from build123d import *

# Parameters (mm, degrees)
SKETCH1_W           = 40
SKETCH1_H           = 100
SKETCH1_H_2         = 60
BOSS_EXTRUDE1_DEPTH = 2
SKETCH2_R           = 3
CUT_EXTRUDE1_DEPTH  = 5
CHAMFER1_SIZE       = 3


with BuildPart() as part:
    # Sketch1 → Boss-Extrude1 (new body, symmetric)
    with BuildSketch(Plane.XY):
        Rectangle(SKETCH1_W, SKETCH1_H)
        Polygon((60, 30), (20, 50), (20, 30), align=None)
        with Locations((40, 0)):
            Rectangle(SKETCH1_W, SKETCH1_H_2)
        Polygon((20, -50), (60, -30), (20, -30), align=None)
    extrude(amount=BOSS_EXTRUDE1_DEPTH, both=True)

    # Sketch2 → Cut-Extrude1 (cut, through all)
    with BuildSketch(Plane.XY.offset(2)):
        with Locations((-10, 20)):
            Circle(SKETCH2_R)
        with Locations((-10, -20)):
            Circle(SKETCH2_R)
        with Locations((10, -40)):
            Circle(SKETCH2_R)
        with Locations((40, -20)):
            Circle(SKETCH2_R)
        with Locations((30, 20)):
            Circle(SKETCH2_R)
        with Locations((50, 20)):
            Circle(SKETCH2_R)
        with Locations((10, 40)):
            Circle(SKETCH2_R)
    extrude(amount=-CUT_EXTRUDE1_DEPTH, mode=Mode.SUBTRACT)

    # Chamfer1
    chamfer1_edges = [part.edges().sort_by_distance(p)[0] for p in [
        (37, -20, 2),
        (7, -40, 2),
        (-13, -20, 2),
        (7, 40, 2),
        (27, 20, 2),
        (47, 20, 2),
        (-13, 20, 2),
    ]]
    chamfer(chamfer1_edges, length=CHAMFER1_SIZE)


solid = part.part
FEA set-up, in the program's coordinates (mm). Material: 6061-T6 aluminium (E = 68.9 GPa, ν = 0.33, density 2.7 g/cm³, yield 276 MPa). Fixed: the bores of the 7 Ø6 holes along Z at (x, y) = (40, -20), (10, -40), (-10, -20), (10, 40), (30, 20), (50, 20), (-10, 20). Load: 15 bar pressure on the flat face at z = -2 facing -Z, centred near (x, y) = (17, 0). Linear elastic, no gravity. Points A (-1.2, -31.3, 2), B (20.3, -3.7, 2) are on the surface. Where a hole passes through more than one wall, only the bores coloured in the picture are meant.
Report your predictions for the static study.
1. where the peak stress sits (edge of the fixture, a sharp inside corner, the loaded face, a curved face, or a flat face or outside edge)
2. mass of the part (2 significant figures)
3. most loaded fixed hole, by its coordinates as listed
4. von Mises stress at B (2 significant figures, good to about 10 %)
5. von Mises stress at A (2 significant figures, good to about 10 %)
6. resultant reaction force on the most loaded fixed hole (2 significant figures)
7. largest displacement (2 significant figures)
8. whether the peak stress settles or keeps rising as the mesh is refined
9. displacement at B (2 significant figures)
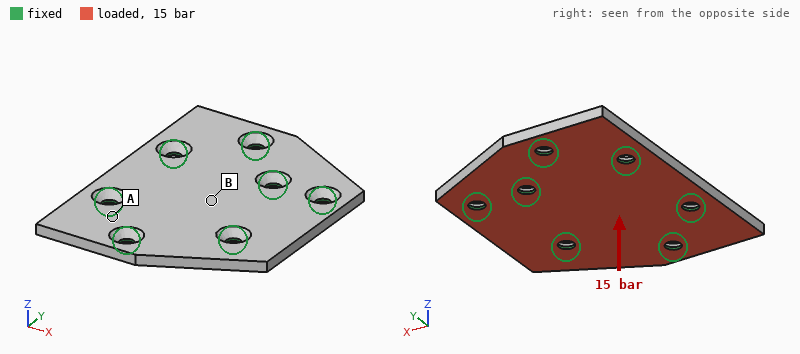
edge of the fixture
73 g
(40, -20)
45 MPa
87 MPa
2.2 kN
0.18 mm
keeps rising
0.072 mm
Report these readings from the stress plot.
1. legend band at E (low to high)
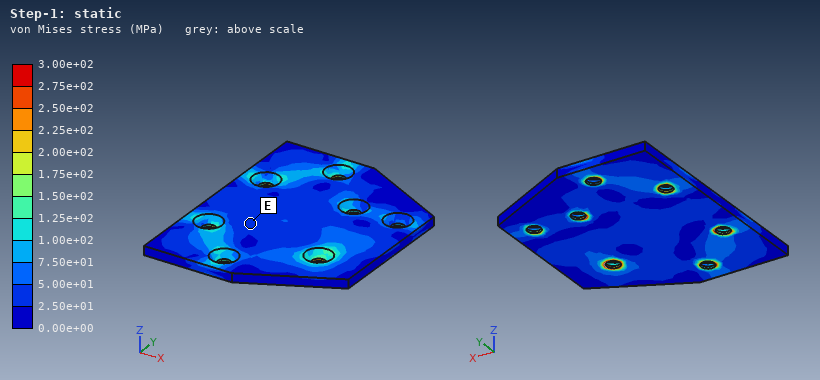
2.50e+01 to 5.00e+01 MPa
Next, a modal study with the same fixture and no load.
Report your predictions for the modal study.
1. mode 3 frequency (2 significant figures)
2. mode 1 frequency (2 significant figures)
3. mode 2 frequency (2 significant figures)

6700 Hz
5500 Hz
5600 Hz
